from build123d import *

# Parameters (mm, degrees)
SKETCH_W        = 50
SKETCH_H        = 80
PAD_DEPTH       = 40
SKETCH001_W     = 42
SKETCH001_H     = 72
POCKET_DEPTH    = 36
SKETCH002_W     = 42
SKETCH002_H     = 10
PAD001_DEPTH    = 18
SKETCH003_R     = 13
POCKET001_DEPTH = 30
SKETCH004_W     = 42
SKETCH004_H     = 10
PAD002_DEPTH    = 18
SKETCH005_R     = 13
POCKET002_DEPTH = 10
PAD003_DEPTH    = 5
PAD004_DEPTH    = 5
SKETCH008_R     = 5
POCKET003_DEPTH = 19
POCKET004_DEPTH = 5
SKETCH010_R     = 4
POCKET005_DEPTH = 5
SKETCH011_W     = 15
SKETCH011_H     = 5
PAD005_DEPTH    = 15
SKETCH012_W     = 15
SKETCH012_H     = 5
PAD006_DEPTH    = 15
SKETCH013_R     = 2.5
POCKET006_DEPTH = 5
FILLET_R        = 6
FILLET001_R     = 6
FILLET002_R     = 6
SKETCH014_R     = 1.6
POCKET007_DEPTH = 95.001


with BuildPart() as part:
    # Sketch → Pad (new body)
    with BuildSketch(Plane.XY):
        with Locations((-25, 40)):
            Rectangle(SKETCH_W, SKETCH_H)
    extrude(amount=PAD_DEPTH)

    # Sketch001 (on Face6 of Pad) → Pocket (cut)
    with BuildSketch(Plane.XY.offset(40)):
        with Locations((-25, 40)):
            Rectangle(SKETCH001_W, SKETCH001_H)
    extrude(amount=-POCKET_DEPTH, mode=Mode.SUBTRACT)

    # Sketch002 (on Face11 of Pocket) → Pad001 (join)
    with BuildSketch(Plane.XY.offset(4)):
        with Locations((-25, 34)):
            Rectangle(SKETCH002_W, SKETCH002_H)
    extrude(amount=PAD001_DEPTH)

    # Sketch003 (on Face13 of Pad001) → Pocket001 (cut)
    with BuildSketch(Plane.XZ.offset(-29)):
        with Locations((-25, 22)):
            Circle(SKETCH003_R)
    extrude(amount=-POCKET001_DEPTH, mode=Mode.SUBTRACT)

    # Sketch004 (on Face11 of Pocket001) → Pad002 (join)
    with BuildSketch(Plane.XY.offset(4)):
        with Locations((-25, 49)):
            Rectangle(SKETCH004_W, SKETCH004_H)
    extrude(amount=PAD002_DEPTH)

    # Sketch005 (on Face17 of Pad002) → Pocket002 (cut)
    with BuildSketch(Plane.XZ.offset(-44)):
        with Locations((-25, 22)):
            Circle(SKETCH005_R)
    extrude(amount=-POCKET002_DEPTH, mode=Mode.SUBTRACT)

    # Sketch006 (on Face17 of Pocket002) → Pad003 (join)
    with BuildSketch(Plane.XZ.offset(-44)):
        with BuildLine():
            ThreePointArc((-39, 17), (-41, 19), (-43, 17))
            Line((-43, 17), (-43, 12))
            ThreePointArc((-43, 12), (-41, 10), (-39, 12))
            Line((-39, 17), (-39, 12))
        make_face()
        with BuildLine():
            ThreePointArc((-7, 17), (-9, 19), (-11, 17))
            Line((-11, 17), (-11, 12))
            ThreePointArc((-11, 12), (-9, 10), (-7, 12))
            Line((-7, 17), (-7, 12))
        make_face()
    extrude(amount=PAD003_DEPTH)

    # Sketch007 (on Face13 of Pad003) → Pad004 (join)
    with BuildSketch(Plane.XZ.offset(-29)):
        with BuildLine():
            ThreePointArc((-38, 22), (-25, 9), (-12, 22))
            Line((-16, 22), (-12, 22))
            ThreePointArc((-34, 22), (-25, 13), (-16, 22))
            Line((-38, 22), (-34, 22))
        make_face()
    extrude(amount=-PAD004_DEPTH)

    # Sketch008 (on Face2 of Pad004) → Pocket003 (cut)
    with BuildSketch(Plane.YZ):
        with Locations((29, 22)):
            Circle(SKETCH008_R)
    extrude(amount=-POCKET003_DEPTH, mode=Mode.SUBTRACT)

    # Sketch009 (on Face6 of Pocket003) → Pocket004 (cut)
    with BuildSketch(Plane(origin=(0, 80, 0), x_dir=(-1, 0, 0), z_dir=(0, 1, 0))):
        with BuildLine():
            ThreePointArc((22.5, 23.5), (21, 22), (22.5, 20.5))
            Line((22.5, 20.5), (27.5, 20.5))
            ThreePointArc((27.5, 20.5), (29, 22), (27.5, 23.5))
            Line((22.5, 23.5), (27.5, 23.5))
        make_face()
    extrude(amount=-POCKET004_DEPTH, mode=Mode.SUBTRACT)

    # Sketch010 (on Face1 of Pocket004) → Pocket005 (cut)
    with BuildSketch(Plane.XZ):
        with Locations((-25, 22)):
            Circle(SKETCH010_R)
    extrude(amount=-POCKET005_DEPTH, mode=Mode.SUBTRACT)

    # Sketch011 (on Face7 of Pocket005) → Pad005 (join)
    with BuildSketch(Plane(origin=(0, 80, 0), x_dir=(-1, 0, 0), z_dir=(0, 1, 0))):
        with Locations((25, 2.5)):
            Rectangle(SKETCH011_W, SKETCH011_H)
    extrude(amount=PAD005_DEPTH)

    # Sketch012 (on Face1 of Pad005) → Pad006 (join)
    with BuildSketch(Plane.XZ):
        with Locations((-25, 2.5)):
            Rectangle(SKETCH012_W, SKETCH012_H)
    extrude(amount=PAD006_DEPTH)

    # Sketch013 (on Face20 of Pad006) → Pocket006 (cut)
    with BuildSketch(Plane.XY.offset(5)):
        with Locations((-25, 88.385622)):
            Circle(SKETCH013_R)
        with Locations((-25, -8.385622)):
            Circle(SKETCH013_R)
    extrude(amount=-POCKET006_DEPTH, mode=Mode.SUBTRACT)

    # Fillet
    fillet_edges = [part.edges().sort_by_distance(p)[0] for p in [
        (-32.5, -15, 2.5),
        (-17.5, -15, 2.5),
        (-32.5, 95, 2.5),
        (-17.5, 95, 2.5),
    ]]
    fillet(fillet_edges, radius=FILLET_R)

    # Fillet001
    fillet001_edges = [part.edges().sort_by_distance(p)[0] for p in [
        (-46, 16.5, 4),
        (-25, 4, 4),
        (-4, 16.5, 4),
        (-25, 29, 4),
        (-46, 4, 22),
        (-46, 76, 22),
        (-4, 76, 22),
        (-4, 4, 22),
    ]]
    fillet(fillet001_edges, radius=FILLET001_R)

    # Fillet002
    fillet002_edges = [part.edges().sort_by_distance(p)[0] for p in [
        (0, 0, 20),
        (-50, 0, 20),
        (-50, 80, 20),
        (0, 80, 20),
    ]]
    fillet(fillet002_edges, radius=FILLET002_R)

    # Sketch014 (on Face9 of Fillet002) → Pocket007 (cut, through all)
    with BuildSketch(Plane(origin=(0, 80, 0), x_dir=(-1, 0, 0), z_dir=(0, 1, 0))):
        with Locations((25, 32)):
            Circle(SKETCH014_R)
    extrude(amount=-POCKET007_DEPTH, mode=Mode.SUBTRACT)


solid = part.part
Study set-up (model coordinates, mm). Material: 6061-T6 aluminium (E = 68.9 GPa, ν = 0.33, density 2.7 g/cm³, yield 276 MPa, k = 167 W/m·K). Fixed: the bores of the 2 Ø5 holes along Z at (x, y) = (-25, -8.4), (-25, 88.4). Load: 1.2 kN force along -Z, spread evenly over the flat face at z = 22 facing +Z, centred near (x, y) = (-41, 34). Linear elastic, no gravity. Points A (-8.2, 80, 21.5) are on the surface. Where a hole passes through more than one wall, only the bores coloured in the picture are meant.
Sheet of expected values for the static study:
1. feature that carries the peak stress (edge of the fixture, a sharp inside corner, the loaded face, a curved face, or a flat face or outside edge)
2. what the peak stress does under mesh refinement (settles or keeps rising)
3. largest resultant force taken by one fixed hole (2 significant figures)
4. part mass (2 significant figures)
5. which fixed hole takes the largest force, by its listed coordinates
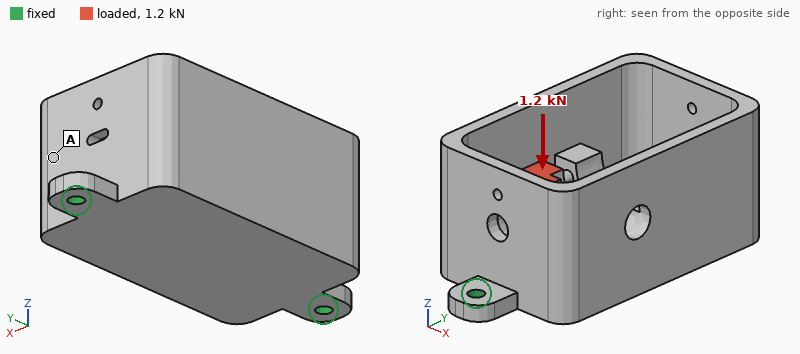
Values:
edge of the fixture
keeps rising
700 N
170 g
(-25, -8.4)
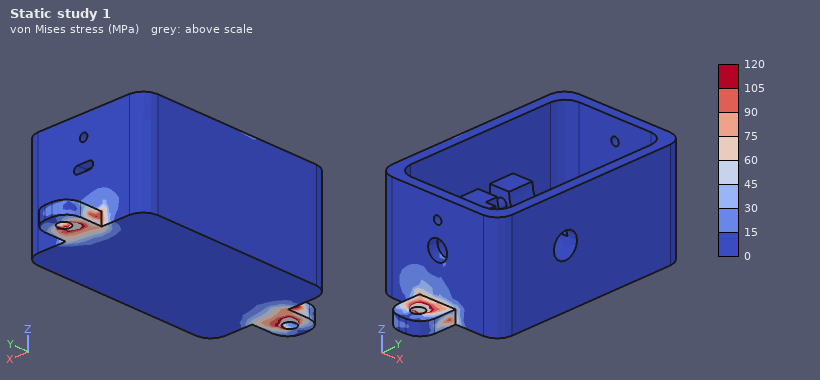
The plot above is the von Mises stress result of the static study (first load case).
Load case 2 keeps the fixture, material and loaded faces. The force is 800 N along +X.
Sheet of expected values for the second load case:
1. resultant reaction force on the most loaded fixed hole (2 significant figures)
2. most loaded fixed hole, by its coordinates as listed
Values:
460 N
(-25, -8.4)
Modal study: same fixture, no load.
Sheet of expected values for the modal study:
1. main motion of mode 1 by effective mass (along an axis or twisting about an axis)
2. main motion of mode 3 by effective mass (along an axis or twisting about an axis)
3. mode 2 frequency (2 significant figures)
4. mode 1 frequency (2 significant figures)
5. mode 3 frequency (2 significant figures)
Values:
along X
along Z
3400 Hz
960 Hz
3600 Hz
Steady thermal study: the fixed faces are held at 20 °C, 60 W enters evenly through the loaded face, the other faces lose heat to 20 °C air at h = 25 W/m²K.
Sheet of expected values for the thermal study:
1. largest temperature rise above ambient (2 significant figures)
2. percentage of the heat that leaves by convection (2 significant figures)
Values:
65 K
29 %
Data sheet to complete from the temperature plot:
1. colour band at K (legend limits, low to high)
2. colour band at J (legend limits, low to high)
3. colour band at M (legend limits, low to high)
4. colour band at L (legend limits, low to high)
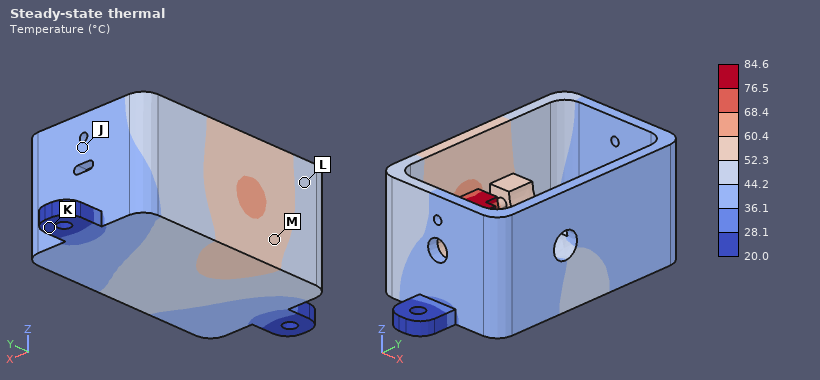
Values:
20.0 to 28.1 °C
36.1 to 44.2 °C
52.3 to 60.4 °C
44.2 to 52.3 °C
